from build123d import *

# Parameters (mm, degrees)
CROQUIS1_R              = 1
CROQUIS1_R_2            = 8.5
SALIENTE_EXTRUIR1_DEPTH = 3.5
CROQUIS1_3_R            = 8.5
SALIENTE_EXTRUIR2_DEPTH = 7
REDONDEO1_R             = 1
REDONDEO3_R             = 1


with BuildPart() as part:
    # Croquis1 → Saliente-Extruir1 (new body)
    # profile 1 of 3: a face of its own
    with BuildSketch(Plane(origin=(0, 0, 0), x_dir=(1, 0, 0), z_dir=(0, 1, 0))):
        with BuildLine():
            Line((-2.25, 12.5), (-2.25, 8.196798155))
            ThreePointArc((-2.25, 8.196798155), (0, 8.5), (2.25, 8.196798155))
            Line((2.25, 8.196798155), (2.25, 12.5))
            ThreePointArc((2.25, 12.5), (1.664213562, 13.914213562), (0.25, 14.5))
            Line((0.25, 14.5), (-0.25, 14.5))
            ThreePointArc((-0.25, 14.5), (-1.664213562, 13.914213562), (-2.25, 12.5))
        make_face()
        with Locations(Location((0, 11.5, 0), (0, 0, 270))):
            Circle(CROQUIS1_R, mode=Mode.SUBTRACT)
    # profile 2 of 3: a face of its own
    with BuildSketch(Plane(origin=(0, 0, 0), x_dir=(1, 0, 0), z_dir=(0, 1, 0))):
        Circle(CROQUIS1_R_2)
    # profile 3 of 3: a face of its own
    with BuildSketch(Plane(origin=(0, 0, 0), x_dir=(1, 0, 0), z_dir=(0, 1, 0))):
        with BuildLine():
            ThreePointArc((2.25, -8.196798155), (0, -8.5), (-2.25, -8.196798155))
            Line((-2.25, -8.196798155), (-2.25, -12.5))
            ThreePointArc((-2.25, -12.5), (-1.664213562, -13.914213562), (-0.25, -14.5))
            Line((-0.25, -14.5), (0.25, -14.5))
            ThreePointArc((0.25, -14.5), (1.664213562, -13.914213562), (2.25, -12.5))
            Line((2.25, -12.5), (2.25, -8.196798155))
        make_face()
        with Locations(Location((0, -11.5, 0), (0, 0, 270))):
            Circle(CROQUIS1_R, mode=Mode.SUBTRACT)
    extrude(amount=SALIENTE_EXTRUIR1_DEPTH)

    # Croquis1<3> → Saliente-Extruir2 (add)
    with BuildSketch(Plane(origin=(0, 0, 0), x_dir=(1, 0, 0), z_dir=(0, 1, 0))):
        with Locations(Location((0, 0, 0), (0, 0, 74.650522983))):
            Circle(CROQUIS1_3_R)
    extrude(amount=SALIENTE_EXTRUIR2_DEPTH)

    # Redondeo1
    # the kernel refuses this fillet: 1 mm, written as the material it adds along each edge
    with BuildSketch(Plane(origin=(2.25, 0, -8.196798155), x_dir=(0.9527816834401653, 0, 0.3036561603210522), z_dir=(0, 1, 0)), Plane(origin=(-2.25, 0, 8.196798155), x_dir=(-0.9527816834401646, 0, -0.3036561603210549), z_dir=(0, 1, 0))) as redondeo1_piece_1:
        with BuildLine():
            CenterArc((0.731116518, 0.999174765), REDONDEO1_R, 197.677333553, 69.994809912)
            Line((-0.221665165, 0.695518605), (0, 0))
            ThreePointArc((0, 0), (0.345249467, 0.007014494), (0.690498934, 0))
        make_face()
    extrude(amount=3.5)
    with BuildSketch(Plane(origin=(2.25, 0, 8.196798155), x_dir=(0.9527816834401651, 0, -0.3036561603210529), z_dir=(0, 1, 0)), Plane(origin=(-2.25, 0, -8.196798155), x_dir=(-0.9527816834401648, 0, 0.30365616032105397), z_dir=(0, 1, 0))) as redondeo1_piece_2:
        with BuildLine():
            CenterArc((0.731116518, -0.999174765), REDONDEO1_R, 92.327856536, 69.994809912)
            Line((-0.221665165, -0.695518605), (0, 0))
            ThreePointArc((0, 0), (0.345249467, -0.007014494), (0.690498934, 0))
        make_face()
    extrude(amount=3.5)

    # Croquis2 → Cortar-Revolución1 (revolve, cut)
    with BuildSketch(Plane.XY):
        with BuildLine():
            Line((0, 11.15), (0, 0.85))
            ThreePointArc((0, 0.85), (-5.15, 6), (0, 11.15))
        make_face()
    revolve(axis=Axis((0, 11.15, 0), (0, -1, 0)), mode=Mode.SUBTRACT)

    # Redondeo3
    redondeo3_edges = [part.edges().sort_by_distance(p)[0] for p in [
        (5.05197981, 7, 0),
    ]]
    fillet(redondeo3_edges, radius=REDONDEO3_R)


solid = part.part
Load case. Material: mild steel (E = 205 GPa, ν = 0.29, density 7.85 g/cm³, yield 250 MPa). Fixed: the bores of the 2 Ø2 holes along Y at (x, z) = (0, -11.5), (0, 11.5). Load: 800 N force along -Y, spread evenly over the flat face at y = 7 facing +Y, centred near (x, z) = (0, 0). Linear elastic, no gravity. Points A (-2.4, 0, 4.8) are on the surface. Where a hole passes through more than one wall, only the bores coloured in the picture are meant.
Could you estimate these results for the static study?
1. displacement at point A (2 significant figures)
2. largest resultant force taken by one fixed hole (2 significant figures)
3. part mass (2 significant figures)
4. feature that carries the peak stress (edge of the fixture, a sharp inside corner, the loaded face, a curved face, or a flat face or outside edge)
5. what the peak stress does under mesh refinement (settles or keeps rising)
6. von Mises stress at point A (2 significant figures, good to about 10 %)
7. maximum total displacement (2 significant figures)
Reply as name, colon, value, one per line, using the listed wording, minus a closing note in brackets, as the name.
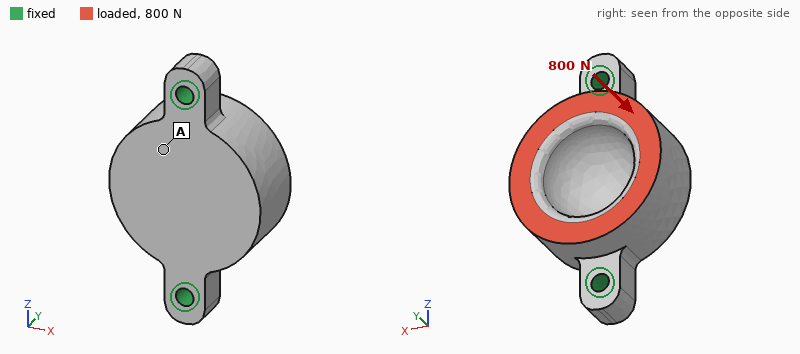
displacement at point A: 3.4 µm
largest resultant force taken by one fixed hole: 400 N
part mass: 11 g
feature that carries the peak stress: edge of the fixture
what the peak stress does under mesh refinement: keeps rising
von Mises stress at point A: 27 MPa
maximum total displacement: 5.8 µm
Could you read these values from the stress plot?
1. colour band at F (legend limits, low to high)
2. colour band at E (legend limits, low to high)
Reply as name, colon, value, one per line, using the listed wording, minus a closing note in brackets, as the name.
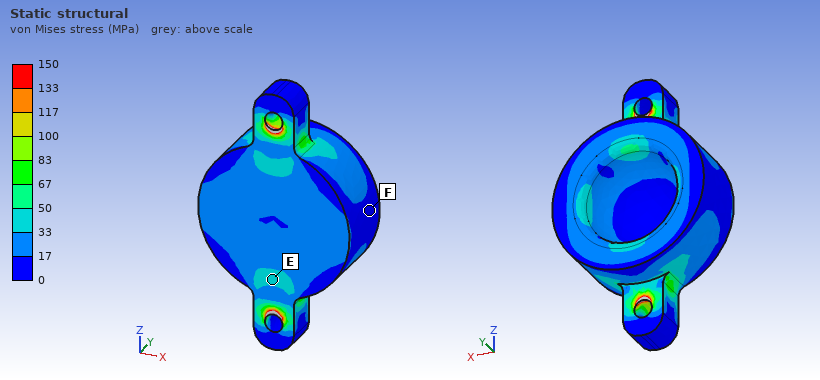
colour band at F: 0 to 17 MPa
colour band at E: 33 to 50 MPa
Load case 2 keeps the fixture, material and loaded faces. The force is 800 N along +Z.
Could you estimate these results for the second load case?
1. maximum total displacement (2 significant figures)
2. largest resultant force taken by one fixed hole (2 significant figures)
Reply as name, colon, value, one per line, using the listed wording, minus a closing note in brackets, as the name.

maximum total displacement: 2.1 µm
largest resultant force taken by one fixed hole: 450 N
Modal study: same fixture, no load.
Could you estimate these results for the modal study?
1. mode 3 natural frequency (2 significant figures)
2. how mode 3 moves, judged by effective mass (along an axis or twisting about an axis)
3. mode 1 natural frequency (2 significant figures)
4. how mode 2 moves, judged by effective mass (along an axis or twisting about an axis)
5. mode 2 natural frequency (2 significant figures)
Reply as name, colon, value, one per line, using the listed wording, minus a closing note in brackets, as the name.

mode 3 natural frequency: 33 kHz
how mode 3 moves, judged by effective mass: along X
mode 1 natural frequency: 12 kHz
how mode 2 moves, judged by effective mass: along Y
mode 2 natural frequency: 22 kHz
